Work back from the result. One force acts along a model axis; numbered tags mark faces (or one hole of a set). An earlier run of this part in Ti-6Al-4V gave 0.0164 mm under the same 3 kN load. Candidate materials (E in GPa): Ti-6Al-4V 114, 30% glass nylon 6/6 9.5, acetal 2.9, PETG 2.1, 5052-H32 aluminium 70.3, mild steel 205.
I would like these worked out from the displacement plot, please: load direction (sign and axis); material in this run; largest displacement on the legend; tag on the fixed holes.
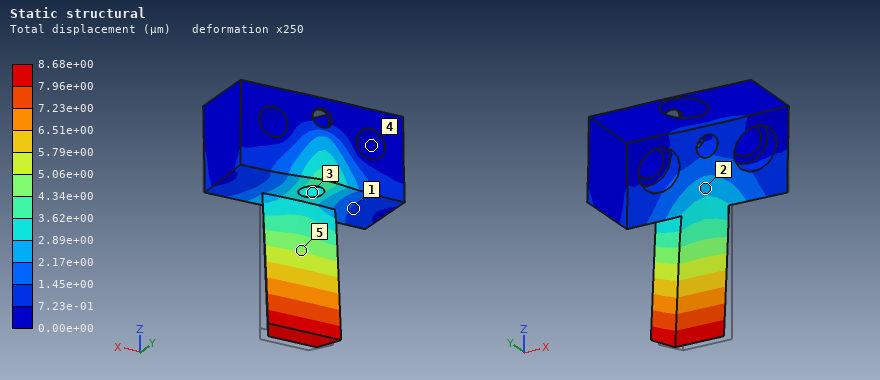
+Y
mild steel
8.68e+00 µm
4
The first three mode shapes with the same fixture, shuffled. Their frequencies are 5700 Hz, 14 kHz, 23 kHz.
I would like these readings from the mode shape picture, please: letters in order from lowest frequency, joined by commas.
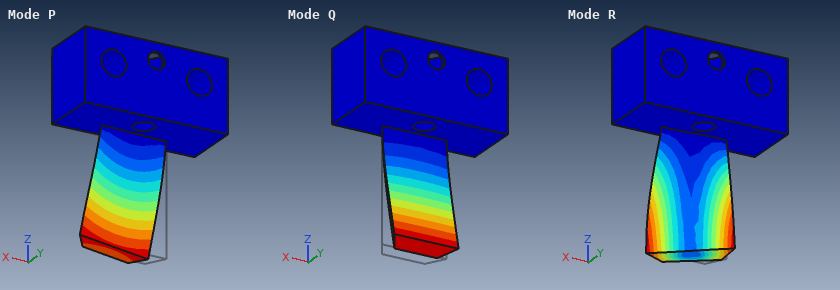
Q, P, R
